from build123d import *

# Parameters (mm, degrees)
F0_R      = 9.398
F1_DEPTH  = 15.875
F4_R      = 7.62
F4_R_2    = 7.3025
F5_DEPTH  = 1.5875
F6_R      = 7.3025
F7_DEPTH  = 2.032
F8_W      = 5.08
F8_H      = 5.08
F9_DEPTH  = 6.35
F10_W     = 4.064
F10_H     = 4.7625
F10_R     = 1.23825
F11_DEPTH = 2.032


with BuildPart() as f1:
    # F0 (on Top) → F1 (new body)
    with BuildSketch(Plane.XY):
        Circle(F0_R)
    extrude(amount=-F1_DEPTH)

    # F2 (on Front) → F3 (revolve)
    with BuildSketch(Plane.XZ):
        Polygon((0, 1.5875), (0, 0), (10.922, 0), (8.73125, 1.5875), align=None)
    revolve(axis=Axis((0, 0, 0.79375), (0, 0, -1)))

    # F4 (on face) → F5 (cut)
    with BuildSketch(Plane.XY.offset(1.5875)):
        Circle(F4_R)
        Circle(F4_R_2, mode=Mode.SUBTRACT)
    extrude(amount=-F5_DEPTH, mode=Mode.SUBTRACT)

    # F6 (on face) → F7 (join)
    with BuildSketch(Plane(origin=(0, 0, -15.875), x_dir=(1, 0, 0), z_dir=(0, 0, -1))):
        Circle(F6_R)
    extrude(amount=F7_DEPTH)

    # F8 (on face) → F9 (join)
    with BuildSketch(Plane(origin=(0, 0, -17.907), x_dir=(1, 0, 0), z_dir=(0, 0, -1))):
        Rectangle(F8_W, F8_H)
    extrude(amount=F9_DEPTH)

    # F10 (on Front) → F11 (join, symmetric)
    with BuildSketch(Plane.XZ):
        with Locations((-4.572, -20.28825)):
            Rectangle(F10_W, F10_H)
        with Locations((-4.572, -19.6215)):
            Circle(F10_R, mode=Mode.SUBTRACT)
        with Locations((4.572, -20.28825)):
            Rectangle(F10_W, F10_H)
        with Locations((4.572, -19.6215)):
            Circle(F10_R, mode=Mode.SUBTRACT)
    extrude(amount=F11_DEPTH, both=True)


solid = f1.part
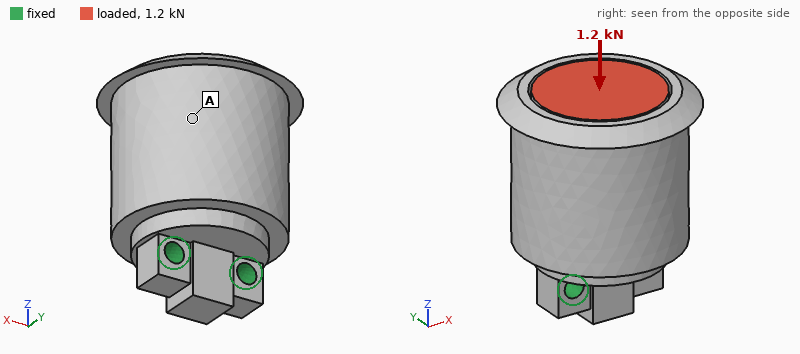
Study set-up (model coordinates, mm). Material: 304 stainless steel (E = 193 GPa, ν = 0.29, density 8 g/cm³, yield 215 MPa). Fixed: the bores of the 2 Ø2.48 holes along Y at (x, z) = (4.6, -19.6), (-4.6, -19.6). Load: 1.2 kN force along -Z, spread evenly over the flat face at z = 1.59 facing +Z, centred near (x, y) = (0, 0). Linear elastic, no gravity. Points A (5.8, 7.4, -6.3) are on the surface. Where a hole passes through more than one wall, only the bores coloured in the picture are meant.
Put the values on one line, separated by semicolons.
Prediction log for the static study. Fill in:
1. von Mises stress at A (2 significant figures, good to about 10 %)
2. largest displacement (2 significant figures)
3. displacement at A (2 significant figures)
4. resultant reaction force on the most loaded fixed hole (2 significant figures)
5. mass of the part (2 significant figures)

3.4 MPa; 1.0 µm; 0.72 µm; 600 N; 44 g
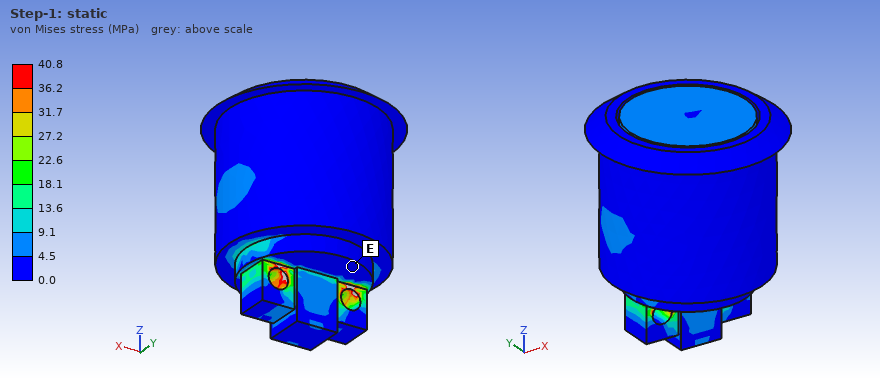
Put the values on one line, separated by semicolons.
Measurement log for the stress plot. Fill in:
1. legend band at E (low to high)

0.0 to 4.5 MPa
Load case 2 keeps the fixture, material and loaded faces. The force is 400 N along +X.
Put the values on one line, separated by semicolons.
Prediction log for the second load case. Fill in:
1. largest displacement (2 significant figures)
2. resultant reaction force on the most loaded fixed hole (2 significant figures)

4.9 µm; 860 N
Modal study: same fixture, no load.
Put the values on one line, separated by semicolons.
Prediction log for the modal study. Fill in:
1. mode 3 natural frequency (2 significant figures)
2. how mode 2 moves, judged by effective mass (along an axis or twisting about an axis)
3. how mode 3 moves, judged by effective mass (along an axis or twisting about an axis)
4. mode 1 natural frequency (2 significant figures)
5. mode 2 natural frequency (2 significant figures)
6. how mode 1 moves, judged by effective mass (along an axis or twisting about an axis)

18 kHz; along X; twisting about Z; 4600 Hz; 12 kHz; along Y
